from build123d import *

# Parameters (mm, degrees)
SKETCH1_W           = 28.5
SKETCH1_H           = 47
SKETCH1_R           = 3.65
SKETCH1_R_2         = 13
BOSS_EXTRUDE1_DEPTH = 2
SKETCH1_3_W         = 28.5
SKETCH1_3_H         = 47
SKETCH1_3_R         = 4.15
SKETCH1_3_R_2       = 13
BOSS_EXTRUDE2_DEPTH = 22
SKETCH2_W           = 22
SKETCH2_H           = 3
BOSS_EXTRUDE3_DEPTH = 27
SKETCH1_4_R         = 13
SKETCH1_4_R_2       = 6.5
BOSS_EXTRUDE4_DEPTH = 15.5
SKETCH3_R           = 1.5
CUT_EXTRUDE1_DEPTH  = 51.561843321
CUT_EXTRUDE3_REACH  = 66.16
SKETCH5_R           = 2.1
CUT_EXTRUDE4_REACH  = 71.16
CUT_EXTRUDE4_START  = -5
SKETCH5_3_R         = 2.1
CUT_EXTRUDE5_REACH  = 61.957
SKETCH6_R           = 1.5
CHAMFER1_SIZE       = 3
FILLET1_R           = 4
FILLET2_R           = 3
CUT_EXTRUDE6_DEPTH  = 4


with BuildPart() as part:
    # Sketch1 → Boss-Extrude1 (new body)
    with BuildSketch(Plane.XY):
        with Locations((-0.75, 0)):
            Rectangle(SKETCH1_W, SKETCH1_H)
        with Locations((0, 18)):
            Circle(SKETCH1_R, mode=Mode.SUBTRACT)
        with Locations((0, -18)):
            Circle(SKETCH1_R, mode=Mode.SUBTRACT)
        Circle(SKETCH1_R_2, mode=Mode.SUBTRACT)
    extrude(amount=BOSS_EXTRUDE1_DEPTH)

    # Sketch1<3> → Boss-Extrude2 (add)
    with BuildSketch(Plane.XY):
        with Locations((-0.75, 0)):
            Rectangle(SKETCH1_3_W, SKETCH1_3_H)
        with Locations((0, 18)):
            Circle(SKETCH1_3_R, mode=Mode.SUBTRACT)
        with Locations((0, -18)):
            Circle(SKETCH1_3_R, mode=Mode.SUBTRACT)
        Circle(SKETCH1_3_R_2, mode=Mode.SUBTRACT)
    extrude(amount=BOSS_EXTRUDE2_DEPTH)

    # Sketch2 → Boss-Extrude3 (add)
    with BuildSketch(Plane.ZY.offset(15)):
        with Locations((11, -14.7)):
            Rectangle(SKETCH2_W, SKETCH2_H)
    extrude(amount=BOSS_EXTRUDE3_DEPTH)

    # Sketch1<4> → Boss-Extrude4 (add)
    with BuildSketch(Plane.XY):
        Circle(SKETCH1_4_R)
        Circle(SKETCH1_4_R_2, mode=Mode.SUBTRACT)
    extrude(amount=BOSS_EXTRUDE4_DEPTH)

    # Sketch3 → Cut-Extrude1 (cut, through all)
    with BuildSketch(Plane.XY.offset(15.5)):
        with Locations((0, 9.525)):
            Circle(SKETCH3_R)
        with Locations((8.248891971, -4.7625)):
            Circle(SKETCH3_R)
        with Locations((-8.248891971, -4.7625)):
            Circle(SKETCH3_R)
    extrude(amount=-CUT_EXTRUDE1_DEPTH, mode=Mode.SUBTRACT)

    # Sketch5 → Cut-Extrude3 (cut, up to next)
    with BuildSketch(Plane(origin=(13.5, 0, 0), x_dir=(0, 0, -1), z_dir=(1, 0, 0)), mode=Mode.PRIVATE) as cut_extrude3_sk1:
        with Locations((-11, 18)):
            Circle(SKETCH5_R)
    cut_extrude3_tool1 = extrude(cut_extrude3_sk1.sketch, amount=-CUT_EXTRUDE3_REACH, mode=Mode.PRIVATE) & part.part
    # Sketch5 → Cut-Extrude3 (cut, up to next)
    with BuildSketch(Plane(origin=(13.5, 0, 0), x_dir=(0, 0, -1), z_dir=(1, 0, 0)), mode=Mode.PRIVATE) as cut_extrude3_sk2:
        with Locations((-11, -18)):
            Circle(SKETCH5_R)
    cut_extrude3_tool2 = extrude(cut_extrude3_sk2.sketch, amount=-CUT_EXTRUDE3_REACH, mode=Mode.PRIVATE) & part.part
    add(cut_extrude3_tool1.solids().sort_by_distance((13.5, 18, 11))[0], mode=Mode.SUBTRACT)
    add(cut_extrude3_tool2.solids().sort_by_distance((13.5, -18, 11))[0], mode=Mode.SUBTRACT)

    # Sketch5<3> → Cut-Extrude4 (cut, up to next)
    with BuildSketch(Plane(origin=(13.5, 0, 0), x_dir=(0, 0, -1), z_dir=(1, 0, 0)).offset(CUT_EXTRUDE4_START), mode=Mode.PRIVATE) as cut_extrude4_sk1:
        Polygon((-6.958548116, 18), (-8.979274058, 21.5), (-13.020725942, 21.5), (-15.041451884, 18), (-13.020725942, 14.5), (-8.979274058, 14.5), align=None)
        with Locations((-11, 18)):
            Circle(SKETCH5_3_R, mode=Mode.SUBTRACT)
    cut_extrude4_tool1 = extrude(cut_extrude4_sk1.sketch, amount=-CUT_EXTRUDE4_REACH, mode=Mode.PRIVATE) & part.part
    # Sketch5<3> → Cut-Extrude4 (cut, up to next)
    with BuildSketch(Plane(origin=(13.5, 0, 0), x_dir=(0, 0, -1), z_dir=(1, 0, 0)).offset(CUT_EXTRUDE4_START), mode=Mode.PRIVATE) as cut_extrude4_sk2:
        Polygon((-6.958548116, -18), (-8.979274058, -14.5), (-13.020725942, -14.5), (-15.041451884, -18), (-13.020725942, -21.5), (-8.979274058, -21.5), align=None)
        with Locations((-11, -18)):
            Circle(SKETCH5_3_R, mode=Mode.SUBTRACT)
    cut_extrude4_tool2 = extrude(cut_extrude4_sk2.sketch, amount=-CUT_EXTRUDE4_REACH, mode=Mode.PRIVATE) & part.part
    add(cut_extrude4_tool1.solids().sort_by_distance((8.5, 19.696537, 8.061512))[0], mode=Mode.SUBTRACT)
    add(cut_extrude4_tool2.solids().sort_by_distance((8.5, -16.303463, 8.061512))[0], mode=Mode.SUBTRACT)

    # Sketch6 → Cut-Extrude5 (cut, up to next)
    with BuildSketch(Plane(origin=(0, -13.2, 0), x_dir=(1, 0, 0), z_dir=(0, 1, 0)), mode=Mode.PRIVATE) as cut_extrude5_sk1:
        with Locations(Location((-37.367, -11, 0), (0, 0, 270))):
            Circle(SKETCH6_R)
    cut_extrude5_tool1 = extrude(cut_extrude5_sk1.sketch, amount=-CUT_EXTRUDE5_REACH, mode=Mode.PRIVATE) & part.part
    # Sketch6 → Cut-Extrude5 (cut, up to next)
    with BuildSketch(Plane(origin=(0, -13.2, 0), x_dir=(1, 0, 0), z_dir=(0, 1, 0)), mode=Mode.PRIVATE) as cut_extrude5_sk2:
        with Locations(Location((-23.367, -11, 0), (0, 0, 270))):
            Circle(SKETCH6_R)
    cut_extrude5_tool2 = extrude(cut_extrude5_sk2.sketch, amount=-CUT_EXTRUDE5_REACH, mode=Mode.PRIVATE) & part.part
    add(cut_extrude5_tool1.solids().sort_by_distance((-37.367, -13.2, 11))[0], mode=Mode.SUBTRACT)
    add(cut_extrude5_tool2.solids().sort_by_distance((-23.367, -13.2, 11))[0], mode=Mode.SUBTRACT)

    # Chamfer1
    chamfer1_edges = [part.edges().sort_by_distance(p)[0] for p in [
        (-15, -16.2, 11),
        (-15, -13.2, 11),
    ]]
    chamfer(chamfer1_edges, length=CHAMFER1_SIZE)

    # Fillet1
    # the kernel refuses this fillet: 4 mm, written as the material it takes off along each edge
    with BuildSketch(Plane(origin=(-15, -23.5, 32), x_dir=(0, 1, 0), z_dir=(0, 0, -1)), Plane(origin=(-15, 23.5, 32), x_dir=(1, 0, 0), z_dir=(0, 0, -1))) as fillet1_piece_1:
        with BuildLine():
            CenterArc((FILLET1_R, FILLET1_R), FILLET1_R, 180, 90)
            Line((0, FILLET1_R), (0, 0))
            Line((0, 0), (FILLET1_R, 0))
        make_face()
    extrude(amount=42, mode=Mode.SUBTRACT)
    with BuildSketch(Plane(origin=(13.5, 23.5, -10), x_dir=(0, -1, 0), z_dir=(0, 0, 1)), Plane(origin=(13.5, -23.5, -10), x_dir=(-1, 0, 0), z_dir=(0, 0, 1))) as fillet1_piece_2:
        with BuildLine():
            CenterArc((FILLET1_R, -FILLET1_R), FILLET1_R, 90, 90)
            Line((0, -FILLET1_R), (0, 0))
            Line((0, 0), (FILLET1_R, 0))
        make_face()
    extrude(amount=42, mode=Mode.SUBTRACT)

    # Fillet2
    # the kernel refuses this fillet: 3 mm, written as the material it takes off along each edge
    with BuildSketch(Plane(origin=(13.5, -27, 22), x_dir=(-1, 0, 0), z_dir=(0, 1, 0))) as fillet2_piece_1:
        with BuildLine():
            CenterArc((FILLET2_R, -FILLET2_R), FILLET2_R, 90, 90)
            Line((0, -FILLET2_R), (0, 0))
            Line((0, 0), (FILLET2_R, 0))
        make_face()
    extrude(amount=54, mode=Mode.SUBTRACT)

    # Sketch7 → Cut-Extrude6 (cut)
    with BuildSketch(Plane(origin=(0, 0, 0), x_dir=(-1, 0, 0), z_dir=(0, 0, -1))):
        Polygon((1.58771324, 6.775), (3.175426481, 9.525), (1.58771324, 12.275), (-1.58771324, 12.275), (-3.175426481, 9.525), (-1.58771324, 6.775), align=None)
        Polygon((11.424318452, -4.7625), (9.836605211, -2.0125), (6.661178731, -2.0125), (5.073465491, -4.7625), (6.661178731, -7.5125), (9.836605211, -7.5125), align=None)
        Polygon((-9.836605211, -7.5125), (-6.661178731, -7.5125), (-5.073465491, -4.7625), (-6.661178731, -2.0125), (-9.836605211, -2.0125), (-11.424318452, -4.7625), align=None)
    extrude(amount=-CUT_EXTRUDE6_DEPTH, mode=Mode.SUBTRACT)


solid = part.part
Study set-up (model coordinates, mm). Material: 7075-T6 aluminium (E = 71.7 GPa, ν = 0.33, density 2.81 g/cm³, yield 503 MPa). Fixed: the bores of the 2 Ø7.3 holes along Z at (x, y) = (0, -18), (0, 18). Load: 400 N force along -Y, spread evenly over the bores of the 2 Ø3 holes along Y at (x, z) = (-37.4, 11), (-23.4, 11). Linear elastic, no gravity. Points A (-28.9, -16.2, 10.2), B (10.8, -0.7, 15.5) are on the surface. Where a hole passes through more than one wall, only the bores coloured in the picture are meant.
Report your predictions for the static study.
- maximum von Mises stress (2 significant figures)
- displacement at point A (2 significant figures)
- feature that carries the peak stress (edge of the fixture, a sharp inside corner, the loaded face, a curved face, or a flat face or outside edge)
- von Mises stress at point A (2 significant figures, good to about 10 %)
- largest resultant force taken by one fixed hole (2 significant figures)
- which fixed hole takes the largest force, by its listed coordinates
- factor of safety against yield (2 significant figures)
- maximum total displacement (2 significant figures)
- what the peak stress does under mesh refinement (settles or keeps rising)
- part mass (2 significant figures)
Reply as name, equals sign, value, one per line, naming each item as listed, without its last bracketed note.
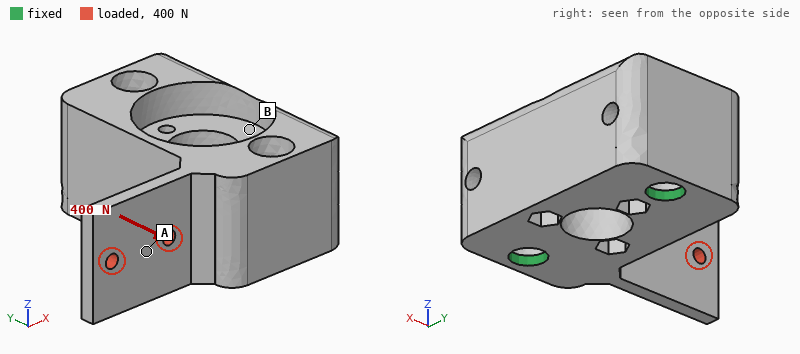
maximum von Mises stress = 160 MPa
displacement at point A = 0.094 mm
feature that carries the peak stress = the loaded face
von Mises stress at point A = 51 MPa
largest resultant force taken by one fixed hole = 380 N
which fixed hole takes the largest force, by its listed coordinates = (0, 18)
factor of safety against yield = 3.1
maximum total displacement = 0.27 mm
what the peak stress does under mesh refinement = settles
part mass = 62 g
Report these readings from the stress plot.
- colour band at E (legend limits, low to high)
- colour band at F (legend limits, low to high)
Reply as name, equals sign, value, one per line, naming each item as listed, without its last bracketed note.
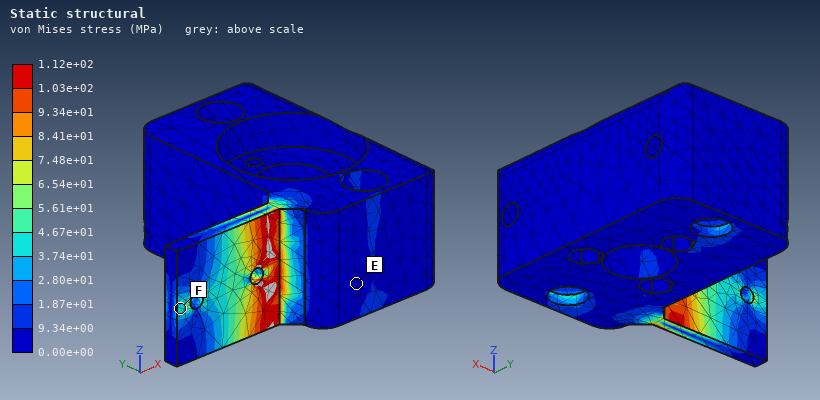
colour band at E = 0.00e+00 to 9.34e+00 MPa
colour band at F = 3.74e+01 to 4.67e+01 MPa
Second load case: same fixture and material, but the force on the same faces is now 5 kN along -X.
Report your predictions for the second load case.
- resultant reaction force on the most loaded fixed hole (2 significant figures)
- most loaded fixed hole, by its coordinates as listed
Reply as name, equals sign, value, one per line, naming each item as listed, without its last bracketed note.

resultant reaction force on the most loaded fixed hole = 4.4 kN
most loaded fixed hole, by its coordinates as listed = (0, -18)
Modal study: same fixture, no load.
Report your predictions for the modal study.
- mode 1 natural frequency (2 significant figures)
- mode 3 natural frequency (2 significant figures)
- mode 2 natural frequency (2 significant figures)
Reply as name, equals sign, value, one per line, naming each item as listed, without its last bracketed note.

mode 1 natural frequency = 3800 Hz
mode 3 natural frequency = 9600 Hz
mode 2 natural frequency = 3800 Hz
